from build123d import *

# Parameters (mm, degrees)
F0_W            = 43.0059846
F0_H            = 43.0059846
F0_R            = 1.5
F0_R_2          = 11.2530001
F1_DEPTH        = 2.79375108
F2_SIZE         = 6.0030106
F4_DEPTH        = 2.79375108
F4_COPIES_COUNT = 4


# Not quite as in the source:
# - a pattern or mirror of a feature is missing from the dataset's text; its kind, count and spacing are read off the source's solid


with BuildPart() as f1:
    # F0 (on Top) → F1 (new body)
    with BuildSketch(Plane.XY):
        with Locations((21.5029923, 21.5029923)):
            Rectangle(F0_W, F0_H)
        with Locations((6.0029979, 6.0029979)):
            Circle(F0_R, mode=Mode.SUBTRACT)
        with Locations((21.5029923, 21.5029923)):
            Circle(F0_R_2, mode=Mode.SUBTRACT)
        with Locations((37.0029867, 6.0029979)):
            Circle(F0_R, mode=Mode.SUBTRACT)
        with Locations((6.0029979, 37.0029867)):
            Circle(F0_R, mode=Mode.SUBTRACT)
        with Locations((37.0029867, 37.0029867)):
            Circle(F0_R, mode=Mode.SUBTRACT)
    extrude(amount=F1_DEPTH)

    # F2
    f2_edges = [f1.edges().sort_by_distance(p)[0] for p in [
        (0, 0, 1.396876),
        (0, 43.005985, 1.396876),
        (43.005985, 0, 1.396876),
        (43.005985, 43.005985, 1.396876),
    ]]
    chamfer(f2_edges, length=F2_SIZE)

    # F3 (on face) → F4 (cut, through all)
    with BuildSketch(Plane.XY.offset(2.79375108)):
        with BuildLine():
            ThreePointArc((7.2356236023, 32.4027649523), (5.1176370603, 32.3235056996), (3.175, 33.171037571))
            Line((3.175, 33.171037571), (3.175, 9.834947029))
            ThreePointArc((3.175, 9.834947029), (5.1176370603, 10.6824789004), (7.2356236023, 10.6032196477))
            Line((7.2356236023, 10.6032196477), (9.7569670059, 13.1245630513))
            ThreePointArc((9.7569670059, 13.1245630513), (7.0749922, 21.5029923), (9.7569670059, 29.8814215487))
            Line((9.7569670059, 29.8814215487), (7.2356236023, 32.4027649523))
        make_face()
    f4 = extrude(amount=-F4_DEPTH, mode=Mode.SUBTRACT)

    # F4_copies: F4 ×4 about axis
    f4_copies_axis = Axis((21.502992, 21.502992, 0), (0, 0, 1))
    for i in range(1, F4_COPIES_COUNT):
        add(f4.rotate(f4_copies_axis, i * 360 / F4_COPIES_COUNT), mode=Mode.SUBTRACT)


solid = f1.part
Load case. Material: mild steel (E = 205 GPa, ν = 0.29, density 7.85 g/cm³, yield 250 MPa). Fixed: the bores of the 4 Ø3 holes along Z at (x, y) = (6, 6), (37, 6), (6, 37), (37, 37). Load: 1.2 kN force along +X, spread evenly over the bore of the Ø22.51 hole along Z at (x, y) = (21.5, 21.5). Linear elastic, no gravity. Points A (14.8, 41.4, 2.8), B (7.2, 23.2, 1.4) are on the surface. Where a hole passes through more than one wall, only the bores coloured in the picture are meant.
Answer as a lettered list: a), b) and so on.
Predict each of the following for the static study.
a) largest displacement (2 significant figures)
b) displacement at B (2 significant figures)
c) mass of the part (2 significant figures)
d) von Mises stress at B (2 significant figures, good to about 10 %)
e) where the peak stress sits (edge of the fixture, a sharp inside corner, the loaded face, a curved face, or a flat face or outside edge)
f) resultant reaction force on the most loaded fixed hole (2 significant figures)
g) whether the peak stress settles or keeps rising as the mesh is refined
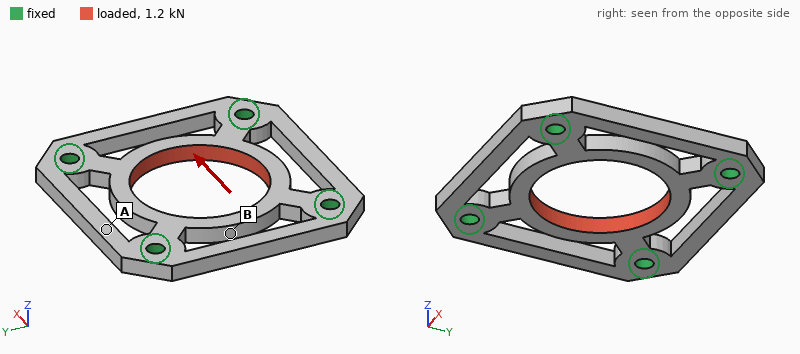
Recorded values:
a) 9.7 µm
b) 9.3 µm
c) 20 g
d) 60 MPa
e) a sharp inside corner
f) 300 N
g) keeps rising
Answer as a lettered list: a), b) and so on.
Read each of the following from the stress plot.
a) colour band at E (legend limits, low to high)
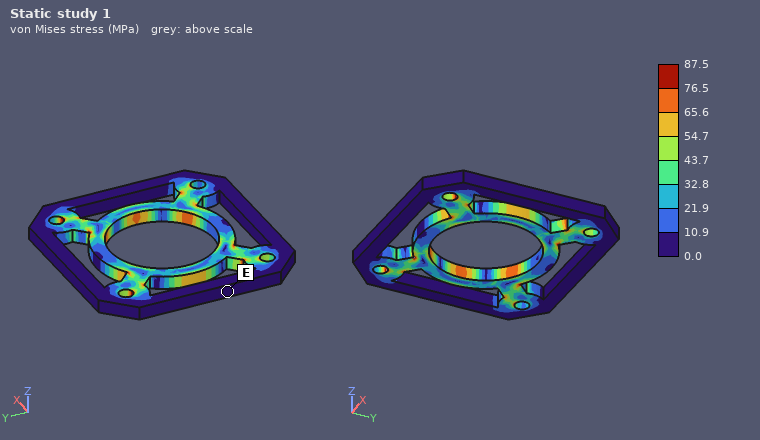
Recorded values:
a) 0.0 to 10.9 MPa
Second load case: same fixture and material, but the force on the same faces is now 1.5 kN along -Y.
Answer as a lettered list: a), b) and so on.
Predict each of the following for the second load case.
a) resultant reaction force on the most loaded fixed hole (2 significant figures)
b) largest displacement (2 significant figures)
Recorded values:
a) 380 N
b) 12 µm
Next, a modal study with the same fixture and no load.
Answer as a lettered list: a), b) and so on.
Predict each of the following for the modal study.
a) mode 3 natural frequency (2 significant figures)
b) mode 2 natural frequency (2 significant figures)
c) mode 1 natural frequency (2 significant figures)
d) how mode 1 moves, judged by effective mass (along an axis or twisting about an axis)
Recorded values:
a) 16 kHz
b) 15 kHz
c) 14 kHz
d) along Z
